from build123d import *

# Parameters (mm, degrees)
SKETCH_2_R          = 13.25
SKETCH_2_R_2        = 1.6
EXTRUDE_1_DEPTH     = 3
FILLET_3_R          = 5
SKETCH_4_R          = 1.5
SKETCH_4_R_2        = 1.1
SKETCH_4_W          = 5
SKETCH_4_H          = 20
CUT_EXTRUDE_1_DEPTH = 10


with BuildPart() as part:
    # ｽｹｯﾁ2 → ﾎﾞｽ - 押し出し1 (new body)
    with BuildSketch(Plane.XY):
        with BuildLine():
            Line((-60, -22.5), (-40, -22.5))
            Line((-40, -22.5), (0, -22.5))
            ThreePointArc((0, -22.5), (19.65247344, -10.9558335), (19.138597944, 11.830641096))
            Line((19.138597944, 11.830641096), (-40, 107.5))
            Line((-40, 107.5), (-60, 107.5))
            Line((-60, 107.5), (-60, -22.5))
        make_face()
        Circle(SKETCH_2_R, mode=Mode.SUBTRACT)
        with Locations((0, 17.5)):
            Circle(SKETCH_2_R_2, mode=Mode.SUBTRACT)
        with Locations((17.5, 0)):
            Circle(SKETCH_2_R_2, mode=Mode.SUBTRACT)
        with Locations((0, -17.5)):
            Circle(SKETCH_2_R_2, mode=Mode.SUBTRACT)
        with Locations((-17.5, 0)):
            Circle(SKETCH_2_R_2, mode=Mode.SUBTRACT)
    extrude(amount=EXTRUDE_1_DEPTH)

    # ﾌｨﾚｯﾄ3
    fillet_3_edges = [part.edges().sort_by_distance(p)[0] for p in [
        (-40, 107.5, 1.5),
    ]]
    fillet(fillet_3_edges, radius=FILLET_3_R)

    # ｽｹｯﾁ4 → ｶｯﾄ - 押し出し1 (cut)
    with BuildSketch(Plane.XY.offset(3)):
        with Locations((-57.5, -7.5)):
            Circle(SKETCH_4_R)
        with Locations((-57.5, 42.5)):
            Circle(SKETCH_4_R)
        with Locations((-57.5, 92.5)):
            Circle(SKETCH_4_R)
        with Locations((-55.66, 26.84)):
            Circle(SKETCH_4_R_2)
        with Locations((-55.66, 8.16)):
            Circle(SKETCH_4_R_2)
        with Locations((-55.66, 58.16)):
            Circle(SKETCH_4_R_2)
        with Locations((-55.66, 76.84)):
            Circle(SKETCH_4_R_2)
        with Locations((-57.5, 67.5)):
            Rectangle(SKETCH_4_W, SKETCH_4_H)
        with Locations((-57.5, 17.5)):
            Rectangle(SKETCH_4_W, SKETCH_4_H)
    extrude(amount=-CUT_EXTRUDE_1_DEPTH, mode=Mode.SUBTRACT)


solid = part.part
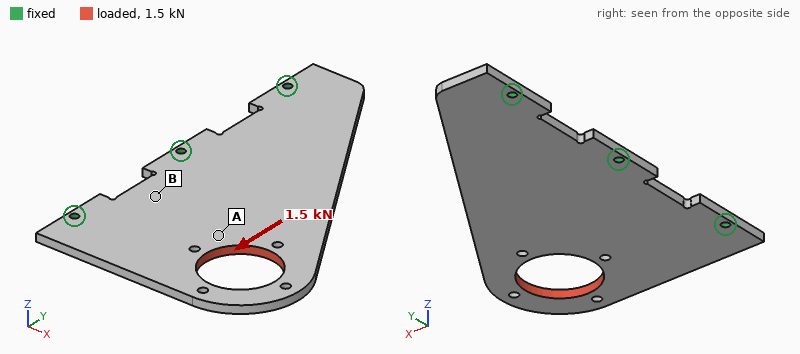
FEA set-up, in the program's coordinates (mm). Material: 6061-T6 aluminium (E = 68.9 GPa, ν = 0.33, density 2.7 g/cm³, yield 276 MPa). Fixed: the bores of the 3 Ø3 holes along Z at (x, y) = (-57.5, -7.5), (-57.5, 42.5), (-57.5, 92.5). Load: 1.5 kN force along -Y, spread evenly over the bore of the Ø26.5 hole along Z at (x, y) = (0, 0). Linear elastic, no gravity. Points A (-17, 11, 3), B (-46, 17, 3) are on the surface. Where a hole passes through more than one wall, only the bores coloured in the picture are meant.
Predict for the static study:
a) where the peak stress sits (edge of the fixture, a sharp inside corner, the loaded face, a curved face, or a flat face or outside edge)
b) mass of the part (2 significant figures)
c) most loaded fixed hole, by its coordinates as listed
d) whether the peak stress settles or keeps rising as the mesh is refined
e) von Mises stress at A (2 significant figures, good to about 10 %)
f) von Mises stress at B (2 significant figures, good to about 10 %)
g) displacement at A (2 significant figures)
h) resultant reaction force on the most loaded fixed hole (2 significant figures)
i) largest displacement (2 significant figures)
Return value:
edge of the fixture
54 g
(-57.5, -7.5)
keeps rising
20 MPa
9.1 MPa
17 µm
1.1 kN
51 µm
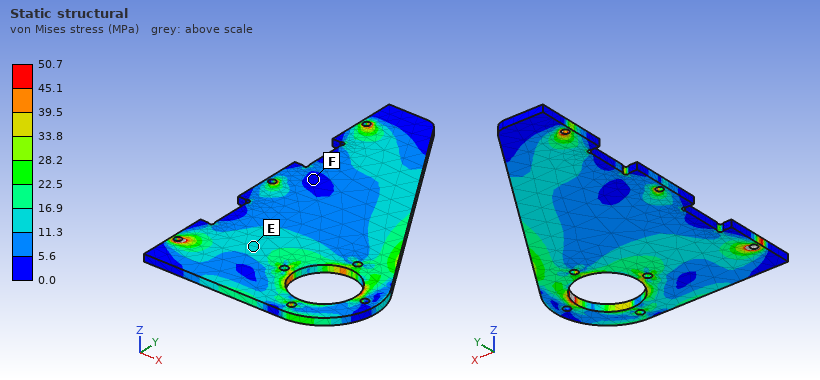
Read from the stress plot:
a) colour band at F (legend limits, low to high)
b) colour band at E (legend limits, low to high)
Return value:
0.0 to 5.6 MPa
11.3 to 16.9 MPa
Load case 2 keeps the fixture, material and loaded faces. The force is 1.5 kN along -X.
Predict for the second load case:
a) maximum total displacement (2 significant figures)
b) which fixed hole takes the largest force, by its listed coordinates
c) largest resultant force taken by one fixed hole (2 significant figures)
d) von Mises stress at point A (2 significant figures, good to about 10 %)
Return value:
29 µm
(-57.5, -7.5)
1.2 kN
12 MPa
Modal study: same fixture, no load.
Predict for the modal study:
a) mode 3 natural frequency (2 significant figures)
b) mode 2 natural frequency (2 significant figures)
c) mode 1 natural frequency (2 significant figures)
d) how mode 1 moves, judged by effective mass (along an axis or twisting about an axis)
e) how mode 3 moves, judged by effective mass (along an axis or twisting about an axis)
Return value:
2200 Hz
1200 Hz
500 Hz
along Z
along Z
